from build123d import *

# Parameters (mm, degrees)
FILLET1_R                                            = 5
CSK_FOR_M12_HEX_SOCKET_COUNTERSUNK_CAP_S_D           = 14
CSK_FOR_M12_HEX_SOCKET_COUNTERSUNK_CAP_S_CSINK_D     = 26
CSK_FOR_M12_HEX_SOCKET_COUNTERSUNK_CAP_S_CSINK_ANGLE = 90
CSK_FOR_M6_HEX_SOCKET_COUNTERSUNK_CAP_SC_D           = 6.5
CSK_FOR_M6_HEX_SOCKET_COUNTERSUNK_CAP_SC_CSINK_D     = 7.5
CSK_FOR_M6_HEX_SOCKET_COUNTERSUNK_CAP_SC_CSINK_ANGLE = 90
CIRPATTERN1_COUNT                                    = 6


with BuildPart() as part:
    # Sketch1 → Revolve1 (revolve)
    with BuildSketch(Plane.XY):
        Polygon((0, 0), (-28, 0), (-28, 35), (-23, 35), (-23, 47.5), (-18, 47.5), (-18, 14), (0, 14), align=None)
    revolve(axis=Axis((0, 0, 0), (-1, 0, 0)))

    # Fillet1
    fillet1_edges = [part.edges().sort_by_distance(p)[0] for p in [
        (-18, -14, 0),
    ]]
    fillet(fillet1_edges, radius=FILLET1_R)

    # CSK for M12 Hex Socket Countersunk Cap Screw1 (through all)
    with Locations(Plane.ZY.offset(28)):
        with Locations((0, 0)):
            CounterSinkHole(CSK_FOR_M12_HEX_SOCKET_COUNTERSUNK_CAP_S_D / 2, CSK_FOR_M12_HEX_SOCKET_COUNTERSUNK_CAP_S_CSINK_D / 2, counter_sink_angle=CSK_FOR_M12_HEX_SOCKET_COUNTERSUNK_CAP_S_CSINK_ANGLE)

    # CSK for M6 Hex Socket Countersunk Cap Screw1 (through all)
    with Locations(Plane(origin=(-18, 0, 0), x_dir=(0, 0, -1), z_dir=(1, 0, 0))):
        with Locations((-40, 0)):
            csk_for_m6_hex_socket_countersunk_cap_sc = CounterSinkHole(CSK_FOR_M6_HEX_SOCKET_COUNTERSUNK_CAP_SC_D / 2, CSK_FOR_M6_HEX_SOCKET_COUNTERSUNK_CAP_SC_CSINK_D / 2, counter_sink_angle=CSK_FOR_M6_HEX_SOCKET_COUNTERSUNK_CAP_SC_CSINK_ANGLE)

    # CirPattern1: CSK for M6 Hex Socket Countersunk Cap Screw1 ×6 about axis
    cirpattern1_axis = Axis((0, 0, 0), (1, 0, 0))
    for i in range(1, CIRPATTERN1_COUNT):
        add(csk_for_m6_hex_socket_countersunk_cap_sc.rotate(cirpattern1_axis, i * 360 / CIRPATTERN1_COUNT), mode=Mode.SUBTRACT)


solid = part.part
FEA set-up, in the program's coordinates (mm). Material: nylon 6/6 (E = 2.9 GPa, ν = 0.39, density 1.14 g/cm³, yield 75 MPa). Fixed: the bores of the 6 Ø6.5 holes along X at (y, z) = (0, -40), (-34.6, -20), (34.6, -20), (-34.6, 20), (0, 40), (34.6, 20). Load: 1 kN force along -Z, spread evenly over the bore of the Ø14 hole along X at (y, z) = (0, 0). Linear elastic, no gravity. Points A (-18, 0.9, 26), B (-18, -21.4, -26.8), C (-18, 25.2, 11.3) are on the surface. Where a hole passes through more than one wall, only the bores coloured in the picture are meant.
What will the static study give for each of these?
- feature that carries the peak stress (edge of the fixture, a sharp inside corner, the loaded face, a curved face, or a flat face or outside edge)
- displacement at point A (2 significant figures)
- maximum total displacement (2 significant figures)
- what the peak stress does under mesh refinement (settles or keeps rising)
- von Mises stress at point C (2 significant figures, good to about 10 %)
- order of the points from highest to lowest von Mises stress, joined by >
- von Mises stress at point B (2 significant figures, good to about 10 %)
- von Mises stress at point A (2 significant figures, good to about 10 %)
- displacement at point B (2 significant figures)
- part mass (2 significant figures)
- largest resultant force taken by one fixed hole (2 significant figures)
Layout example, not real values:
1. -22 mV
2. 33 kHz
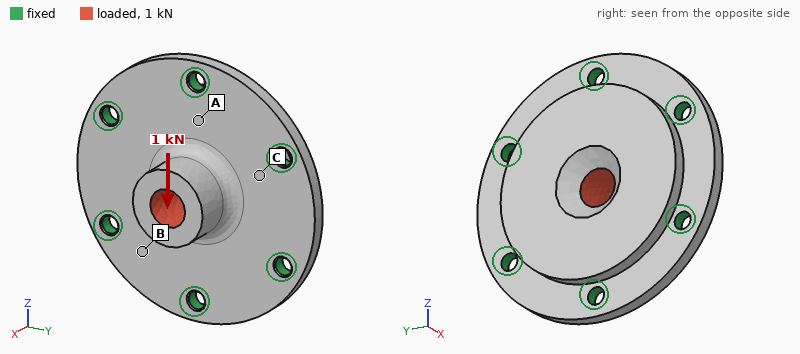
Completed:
1. edge of the fixture
2. 0.026 mm
3. 0.10 mm
4. keeps rising
5. 2.3 MPa
6. A > C > B
7. 0.94 MPa
8. 3.6 MPa
9. 0.017 mm
10. 68 g
11. 240 N
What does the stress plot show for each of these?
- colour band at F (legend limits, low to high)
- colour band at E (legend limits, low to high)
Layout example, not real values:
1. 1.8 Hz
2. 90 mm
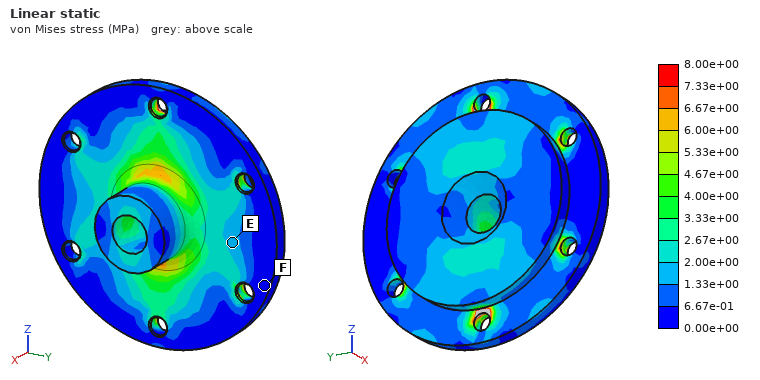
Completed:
1. 0.00e+00 to 6.67e-01 MPa
2. 1.33e+00 to 2.00e+00 MPa
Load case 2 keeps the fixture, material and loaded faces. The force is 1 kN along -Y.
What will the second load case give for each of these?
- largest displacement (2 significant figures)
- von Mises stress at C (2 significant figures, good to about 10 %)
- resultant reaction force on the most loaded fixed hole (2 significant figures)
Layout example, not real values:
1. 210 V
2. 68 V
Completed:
1. 0.10 mm
2. 2.8 MPa
3. 220 N
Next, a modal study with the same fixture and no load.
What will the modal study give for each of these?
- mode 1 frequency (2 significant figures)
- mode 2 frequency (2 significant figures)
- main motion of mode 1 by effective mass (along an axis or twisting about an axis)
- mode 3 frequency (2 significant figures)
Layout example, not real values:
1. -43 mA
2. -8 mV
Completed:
1. 2700 Hz
2. 4200 Hz
3. along X
4. 4200 Hz
